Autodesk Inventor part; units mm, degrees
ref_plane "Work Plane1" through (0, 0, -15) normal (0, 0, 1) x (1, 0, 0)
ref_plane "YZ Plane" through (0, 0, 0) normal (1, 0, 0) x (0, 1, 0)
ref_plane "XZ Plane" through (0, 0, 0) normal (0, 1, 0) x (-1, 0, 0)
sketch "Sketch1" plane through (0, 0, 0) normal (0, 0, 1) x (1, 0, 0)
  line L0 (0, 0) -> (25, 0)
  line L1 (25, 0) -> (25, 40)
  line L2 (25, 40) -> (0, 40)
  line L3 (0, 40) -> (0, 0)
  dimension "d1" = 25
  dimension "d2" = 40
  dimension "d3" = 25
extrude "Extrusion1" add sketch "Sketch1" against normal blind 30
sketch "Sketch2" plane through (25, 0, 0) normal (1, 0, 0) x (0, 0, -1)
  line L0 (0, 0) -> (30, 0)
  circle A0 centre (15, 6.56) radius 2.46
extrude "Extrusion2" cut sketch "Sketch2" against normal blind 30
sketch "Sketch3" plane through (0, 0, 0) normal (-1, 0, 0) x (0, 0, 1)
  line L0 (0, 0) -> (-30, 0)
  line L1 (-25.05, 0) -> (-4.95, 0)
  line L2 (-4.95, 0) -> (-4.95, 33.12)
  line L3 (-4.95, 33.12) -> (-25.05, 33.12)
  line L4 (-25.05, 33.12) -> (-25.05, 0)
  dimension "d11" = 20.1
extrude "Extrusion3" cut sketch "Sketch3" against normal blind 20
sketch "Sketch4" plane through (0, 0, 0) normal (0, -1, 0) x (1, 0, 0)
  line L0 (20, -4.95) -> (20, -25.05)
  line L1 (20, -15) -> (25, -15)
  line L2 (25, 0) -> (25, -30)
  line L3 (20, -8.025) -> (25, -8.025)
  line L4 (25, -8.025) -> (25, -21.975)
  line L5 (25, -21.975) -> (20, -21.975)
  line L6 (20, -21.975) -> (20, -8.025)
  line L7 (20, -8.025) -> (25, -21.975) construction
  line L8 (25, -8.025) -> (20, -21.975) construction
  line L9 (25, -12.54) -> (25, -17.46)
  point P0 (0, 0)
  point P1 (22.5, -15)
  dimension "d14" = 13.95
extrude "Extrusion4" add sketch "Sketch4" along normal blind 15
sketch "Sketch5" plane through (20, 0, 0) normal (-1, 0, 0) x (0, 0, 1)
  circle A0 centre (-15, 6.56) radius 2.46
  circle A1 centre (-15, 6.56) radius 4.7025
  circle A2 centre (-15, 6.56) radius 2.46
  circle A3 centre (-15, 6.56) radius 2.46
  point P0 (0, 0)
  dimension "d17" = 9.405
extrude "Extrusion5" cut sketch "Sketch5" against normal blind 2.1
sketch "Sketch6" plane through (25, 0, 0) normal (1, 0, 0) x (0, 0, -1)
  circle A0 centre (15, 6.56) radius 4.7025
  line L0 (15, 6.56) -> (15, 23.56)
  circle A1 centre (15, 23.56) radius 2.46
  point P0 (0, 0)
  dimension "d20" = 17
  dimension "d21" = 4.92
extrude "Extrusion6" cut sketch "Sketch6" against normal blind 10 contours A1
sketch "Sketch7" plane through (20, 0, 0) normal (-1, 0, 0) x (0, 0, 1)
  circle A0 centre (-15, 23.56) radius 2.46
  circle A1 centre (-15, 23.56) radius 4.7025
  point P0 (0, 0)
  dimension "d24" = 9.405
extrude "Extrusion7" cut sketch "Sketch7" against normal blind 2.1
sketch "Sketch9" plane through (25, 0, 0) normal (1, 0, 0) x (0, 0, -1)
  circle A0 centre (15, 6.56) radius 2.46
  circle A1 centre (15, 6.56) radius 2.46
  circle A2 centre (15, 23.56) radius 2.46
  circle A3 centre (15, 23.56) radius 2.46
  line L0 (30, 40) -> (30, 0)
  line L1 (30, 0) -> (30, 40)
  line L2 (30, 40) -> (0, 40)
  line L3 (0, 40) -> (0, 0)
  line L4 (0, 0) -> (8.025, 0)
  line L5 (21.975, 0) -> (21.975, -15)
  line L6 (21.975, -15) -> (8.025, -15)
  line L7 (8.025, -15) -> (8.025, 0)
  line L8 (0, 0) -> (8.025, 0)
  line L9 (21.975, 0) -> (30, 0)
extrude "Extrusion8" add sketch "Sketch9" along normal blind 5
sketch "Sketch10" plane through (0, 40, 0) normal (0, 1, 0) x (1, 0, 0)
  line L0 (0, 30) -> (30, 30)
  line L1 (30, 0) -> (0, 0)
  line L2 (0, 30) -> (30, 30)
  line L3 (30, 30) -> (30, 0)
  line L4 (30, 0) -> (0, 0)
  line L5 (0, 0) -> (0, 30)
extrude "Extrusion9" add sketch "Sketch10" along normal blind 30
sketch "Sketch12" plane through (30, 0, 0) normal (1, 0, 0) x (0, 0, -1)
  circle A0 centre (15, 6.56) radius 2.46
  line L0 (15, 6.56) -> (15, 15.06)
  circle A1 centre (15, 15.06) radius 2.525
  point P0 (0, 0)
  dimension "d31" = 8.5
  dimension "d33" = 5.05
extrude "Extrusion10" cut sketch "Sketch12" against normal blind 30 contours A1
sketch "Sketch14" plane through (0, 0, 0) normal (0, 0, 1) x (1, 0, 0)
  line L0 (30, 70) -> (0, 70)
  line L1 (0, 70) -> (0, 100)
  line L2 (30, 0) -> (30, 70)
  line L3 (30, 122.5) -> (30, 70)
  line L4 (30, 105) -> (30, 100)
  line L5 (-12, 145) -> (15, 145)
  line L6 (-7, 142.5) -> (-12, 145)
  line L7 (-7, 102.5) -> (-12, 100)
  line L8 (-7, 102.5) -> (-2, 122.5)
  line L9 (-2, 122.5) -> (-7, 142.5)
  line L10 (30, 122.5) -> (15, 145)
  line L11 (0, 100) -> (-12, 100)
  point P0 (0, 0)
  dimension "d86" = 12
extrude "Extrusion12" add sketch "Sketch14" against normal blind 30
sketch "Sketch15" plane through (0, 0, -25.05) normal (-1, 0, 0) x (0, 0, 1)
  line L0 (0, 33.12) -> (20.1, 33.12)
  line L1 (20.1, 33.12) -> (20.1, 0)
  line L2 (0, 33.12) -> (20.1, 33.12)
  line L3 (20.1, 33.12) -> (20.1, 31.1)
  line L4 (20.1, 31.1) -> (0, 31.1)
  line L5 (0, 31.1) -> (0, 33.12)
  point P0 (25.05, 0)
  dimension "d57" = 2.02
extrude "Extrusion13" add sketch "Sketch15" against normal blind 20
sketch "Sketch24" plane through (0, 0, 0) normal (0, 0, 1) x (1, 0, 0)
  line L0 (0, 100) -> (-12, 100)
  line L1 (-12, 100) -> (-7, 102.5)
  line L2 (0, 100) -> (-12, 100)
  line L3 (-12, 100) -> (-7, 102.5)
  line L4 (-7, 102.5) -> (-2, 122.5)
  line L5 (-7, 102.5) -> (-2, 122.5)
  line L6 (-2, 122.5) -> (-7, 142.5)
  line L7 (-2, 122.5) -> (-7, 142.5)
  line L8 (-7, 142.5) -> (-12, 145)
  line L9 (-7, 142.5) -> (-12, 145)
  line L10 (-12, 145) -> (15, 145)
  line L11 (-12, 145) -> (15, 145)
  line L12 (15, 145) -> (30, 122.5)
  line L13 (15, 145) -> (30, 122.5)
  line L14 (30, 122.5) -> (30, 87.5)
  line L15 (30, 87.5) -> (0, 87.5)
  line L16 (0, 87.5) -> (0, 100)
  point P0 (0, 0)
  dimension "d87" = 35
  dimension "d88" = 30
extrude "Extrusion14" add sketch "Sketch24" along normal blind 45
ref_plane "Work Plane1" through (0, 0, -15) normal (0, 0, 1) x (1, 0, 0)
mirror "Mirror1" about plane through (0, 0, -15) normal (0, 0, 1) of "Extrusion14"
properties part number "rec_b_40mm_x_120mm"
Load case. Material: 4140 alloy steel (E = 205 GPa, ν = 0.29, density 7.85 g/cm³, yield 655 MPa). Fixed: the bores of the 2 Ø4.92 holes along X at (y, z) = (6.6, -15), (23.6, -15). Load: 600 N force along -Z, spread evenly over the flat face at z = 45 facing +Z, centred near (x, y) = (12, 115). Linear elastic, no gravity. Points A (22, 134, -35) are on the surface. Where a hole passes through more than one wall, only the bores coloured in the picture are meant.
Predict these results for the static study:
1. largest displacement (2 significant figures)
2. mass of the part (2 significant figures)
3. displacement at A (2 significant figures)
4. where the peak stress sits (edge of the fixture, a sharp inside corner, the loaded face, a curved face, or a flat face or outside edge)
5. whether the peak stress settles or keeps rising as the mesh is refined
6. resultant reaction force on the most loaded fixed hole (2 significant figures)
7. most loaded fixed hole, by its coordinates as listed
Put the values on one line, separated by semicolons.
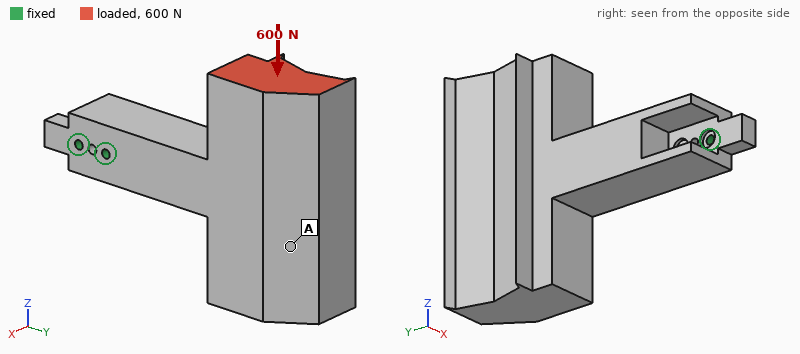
55 µm; 2.2 kg; 43 µm; edge of the fixture; keeps rising; 2.9 kN; (23.6, -15)
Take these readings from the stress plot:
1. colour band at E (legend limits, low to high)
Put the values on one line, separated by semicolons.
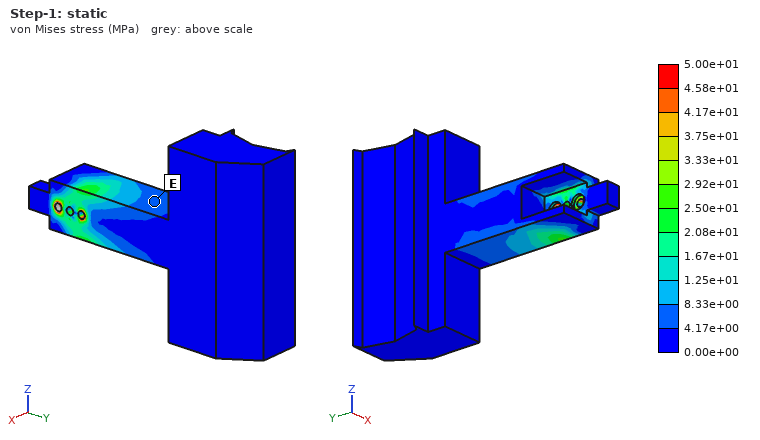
4.17e+00 to 8.33e+00 MPa
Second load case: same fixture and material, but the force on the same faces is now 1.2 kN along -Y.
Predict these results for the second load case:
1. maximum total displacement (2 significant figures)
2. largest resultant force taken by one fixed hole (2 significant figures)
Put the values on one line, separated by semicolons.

90 µm; 3.3 kN
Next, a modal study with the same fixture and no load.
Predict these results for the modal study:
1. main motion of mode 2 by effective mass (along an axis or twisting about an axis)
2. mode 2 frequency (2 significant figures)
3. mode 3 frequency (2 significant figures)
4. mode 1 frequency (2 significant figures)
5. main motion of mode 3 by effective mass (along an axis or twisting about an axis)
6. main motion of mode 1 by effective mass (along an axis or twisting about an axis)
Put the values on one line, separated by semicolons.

along Z; 460 Hz; 710 Hz; 420 Hz; twisting about Y; along X
